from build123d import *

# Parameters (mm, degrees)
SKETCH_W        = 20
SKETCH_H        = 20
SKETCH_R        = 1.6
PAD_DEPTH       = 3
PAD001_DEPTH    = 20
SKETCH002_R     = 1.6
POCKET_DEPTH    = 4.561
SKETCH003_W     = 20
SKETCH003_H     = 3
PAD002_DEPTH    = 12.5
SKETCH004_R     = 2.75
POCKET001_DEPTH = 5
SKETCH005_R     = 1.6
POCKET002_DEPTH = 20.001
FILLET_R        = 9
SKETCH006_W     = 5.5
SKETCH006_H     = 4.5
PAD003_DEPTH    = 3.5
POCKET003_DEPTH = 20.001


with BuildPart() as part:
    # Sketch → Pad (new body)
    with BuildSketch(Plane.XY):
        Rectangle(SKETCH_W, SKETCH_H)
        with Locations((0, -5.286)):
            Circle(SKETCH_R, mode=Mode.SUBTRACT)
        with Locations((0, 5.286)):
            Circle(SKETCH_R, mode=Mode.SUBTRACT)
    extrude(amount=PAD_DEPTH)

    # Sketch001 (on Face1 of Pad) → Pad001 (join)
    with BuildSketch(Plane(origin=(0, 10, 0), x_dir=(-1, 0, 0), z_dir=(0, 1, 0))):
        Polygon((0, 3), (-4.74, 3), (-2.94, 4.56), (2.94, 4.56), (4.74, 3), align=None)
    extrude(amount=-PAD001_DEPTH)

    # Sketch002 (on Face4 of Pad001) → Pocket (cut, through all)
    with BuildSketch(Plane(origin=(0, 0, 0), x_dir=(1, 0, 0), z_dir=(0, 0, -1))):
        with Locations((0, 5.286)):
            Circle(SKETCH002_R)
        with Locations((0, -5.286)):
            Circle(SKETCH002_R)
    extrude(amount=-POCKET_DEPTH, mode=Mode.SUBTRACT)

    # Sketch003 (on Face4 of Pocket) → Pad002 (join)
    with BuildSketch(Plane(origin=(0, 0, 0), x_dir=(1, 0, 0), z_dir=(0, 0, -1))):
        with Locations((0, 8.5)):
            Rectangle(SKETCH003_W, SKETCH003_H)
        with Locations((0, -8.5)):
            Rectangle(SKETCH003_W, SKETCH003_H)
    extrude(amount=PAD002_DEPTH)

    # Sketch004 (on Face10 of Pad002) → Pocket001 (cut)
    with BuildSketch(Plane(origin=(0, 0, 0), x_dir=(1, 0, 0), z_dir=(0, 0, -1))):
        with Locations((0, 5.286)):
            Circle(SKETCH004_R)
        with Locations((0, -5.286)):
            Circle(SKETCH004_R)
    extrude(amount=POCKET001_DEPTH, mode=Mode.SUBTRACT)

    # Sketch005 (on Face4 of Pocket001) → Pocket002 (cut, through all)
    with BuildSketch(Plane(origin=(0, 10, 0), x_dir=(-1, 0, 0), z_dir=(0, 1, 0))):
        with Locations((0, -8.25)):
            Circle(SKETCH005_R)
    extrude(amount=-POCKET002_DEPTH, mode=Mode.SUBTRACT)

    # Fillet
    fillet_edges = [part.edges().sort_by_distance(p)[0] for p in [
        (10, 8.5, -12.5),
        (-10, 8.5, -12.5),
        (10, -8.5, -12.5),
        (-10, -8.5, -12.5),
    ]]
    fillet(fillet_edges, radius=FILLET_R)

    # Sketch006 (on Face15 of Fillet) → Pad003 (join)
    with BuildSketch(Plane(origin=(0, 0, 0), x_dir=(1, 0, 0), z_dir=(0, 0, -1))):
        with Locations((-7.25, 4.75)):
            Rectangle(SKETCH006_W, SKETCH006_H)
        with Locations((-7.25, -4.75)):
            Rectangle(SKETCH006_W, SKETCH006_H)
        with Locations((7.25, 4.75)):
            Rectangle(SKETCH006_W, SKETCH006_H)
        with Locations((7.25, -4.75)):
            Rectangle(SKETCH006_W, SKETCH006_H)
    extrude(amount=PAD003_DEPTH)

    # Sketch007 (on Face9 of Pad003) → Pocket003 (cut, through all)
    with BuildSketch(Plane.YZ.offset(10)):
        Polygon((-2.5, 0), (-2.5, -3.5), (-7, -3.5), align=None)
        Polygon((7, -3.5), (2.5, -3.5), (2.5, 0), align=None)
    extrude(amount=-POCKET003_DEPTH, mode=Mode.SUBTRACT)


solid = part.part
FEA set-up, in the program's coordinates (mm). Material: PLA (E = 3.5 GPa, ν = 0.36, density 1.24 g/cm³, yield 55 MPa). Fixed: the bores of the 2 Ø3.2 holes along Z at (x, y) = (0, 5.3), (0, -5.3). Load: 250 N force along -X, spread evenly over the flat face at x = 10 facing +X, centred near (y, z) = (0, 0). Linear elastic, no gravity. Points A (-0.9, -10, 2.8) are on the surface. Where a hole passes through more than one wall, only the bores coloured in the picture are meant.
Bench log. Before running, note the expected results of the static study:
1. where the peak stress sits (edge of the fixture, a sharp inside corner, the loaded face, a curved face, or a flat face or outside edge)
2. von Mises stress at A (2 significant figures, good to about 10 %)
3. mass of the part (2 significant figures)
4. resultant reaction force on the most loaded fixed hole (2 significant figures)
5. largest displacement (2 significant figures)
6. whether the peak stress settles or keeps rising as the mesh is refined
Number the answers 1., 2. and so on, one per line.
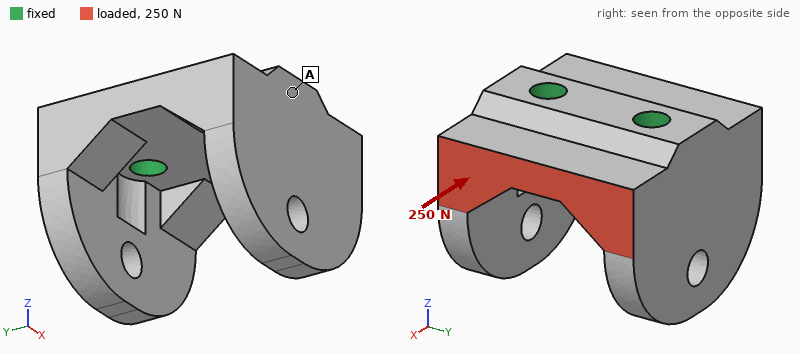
1. edge of the fixture
2. 1.1 MPa
3. 3.4 g
4. 130 N
5. 28 µm
6. keeps rising
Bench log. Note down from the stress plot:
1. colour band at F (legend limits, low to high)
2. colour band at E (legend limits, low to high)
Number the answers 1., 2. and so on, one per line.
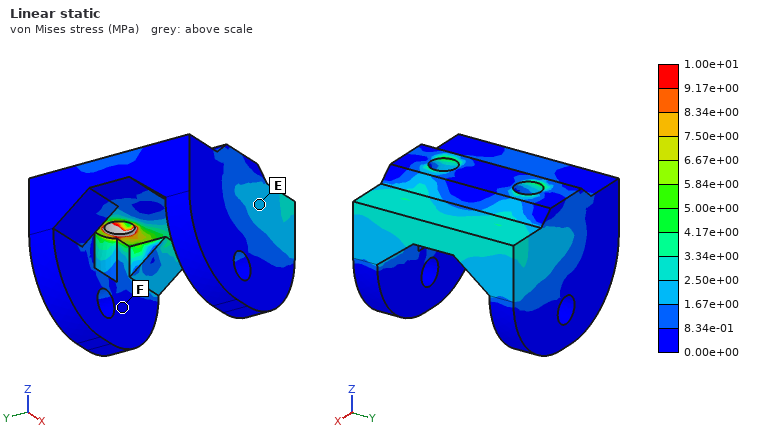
1. 0.00e+00 to 8.34e-01 MPa
2. 1.67e+00 to 2.50e+00 MPa
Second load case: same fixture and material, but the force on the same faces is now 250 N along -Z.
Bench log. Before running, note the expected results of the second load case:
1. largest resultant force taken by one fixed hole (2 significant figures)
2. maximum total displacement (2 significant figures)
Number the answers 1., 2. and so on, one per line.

1. 130 N
2. 0.13 mm
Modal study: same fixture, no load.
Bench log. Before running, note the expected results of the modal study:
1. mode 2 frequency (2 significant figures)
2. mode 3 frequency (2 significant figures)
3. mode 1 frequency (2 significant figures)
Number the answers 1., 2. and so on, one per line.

1. 5700 Hz
2. 5700 Hz
3. 5300 Hz
